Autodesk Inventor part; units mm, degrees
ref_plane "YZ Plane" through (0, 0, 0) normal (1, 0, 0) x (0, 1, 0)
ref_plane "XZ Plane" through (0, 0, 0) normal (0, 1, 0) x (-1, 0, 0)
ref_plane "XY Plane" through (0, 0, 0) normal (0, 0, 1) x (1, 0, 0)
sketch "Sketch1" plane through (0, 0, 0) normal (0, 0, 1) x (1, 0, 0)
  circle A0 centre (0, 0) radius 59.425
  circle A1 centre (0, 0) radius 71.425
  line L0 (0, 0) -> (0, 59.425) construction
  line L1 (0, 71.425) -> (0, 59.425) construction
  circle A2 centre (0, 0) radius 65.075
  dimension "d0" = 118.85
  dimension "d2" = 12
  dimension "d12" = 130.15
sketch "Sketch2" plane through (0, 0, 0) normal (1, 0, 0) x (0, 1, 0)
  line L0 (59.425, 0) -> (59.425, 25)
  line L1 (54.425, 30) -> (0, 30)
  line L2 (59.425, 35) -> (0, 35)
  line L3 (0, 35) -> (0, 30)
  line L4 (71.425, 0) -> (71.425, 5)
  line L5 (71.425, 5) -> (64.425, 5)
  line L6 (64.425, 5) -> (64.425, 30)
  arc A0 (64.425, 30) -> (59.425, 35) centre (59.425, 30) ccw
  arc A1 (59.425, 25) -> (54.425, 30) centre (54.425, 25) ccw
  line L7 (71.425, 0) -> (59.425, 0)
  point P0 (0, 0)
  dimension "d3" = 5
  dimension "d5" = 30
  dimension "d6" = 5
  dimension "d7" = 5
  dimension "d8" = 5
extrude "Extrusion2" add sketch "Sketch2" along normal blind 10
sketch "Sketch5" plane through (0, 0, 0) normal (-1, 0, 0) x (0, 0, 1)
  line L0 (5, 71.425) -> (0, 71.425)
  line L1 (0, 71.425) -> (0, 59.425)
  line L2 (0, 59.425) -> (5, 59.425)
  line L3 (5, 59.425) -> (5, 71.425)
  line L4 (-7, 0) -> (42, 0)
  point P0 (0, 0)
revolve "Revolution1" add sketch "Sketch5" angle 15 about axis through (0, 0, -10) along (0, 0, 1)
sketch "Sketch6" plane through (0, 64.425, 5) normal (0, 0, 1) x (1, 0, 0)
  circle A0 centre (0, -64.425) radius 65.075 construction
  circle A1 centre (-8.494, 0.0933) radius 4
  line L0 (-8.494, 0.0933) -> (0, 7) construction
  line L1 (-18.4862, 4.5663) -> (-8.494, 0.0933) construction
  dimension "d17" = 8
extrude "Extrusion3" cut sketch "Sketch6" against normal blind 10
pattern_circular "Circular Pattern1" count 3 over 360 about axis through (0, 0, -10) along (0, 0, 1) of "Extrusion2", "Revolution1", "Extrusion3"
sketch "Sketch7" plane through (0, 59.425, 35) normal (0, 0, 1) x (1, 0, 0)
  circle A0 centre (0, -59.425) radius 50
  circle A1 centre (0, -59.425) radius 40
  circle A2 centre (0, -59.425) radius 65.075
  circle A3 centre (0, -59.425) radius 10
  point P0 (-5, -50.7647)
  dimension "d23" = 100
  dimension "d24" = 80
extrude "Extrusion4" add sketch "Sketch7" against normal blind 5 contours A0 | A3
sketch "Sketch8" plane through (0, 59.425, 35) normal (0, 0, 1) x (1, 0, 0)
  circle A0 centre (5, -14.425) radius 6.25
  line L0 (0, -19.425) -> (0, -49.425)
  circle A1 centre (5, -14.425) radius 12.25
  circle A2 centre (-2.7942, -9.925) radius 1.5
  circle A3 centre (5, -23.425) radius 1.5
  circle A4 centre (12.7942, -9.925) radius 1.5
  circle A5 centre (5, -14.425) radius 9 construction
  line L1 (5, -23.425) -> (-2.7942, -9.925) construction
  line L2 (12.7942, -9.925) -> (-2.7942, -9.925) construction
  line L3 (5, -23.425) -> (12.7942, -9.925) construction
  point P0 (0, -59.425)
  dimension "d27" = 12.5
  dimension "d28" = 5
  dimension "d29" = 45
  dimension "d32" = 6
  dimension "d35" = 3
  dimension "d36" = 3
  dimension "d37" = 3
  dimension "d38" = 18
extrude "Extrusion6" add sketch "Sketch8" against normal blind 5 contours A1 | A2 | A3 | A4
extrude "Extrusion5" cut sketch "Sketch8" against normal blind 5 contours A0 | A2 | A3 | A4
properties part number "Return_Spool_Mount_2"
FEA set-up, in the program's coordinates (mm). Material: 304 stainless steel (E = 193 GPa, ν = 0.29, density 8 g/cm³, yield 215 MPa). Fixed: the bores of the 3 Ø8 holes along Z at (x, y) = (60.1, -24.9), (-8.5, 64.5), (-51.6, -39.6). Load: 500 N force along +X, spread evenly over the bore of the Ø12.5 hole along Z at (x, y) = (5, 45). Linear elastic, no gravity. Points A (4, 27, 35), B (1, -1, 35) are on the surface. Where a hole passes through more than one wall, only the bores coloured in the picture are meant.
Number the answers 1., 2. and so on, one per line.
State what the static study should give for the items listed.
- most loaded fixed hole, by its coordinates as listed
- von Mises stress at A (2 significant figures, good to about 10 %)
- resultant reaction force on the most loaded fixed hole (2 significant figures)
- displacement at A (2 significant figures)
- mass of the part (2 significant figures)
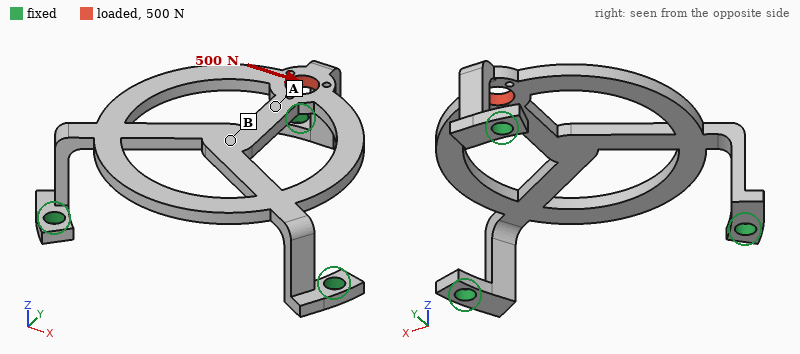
1. (-8.5, 64.5)
2. 29 MPa
3. 280 N
4. 68 µm
5. 240 g
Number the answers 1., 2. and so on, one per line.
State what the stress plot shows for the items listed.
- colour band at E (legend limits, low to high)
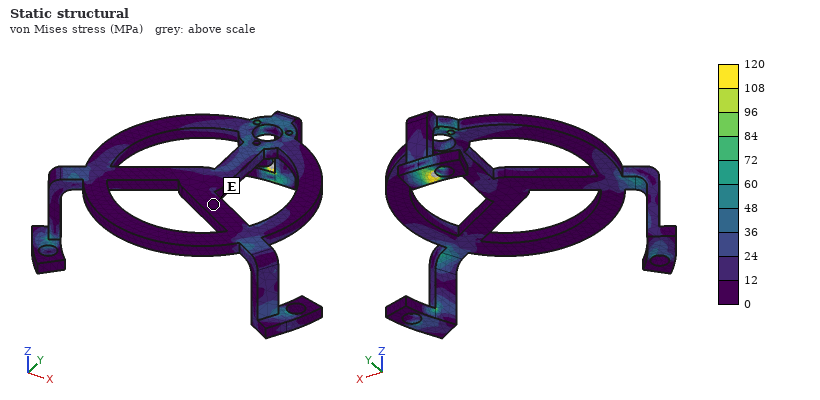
1. 0 to 12 MPa
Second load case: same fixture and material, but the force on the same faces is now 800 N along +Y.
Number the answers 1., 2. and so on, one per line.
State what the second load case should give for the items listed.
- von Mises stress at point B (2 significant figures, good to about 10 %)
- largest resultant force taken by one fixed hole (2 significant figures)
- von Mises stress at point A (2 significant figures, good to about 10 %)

1. 16 MPa
2. 310 N
3. 14 MPa
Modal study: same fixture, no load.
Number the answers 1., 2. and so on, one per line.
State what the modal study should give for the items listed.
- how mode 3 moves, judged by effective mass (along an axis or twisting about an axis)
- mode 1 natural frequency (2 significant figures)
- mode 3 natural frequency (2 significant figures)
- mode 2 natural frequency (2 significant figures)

1. along Z
2. 1200 Hz
3. 1400 Hz
4. 1200 Hz
